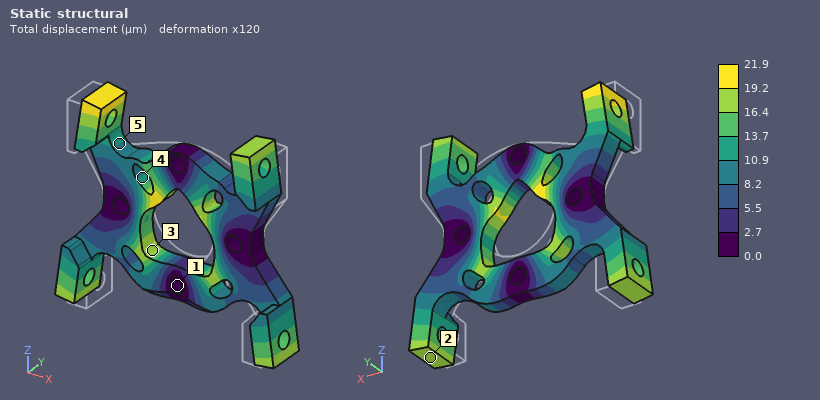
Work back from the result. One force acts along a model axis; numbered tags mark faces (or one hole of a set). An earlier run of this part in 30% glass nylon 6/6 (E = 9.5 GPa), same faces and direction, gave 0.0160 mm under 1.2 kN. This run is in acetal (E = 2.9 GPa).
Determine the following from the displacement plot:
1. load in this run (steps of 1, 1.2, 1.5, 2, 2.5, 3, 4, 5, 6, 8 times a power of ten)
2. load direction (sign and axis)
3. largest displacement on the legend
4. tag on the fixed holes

500 N
-Z
21.9 µm
1
